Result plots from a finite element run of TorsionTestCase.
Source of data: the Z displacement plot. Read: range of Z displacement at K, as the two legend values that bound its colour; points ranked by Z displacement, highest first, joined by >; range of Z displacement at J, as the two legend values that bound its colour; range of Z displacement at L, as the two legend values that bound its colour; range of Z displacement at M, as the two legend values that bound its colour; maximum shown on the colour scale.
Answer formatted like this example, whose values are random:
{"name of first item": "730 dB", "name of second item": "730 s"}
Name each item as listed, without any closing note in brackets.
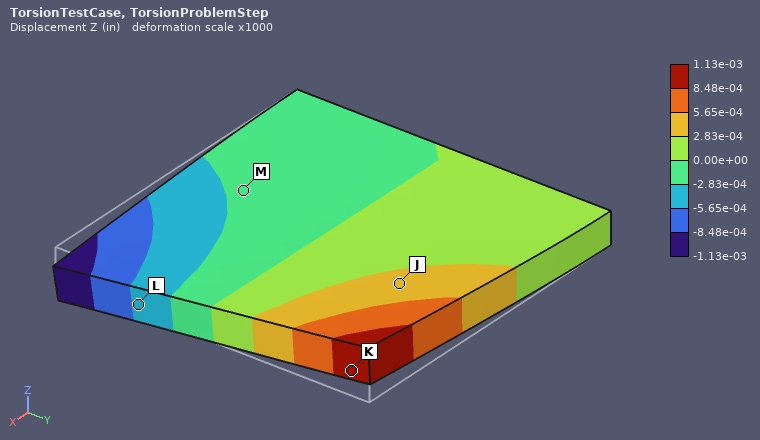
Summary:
{"range of Z displacement at K, as the two legend values that bound its colour": "8.48e-04 to 1.13e-03 in", "points ranked by Z displacement, highest first, joined by >": "K > J > M > L", "range of Z displacement at J, as the two legend values that bound its colour": "2.83e-04 to 5.65e-04 in", "range of Z displacement at L, as the two legend values that bound its colour": "-5.65e-04 to -2.83e-04 in", "range of Z displacement at M, as the two legend values that bound its colour": "-2.83e-04 to 0.00e+00 in", "maximum shown on the colour scale": "1.13e-03 in"}
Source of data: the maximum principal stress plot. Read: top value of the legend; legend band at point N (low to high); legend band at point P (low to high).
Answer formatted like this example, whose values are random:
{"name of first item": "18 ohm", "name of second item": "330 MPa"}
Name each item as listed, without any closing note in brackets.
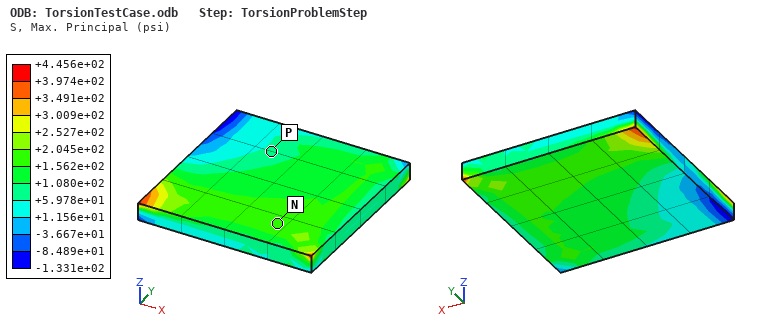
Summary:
{"top value of the legend": "+4.456e+02 psi", "legend band at point N": "+1.562e+02 to +2.045e+02 psi", "legend band at point P": "+5.978e+01 to +1.080e+02 psi"}
